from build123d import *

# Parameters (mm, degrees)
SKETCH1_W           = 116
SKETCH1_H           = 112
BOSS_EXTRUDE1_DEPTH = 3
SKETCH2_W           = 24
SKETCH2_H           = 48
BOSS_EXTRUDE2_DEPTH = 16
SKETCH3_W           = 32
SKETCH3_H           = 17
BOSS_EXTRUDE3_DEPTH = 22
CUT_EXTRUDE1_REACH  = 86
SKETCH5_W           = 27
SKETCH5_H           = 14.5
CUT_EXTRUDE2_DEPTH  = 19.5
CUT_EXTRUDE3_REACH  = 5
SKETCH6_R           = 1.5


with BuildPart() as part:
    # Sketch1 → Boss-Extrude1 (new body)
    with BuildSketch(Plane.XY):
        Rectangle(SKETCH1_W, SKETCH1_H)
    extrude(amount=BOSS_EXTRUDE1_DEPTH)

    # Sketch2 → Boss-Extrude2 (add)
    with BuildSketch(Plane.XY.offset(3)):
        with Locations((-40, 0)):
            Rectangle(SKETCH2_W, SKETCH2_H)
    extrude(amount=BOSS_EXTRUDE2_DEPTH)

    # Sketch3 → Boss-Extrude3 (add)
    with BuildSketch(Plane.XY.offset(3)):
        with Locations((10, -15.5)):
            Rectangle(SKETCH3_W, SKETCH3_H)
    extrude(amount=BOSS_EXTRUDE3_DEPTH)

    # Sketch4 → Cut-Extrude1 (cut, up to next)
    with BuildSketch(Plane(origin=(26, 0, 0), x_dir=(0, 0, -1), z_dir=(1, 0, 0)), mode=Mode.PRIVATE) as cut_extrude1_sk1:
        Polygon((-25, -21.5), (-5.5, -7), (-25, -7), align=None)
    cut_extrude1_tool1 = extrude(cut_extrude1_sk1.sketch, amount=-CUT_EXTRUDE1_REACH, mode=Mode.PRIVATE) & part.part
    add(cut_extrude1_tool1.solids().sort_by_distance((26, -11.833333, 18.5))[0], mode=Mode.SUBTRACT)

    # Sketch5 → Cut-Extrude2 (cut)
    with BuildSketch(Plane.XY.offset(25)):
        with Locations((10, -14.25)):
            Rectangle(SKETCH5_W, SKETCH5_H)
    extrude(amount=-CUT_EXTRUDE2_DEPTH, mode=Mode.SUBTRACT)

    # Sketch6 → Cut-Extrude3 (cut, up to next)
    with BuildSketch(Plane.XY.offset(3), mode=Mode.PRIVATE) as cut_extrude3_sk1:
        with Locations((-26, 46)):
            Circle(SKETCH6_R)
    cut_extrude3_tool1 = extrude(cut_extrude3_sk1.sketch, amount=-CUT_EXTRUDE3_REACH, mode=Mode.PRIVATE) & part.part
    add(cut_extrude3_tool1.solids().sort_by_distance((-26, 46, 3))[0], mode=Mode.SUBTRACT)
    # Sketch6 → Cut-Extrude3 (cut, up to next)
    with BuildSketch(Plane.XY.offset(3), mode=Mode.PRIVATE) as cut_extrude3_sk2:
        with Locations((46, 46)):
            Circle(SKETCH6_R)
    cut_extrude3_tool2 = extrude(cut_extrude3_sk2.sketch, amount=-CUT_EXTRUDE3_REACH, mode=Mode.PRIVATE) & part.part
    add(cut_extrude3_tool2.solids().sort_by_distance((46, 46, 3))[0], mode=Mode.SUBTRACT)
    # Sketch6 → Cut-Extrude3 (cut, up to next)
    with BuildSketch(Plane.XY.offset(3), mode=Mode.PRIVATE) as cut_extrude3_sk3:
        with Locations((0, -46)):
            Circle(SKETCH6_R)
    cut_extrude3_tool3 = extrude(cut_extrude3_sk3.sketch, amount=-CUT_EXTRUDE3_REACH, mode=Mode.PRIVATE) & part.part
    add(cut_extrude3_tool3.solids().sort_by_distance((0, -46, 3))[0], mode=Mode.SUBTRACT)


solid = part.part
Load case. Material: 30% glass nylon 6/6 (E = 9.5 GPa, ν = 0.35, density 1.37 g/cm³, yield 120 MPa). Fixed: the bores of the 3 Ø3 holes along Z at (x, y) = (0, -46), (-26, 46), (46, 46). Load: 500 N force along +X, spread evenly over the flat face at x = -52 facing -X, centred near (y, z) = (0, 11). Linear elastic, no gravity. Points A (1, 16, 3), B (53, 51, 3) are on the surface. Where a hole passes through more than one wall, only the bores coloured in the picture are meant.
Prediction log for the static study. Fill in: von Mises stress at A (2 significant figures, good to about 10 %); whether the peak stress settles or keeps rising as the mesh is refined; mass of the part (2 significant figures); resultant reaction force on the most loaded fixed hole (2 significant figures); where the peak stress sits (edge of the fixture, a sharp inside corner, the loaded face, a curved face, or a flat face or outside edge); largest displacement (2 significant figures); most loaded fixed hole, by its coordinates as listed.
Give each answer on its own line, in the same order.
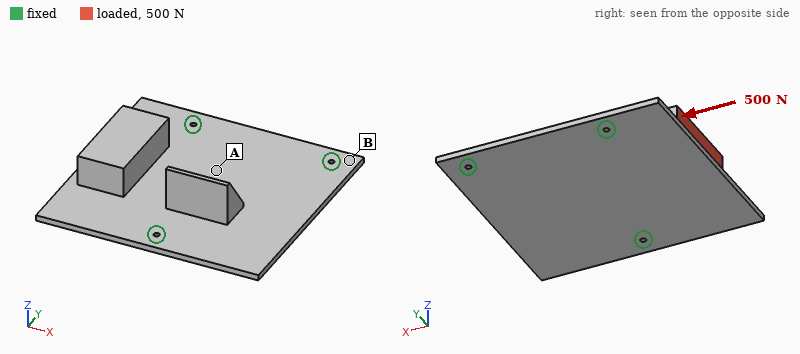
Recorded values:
9.5 MPa
keeps rising
84 g
230 N
edge of the fixture
1.7 mm
(0, -46)
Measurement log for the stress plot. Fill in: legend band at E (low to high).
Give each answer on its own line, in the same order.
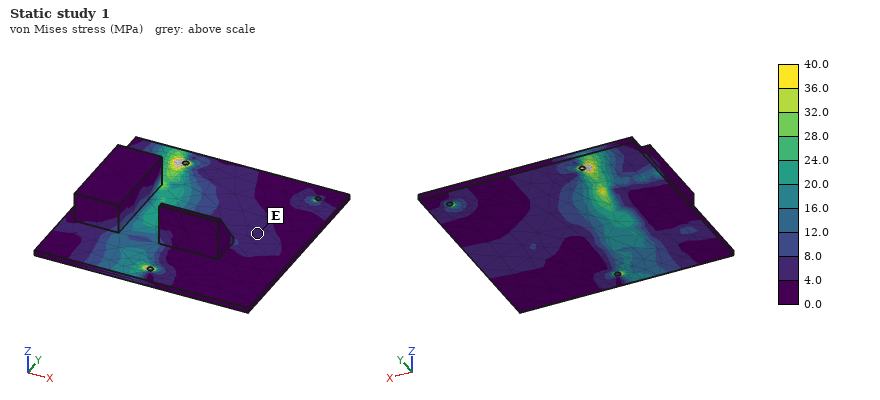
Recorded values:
4.0 to 8.0 MPa
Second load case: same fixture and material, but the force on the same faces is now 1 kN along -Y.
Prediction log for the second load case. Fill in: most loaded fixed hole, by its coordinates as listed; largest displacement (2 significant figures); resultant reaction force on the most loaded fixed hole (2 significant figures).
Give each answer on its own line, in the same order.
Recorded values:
(-26, 46)
1.6 mm
680 N
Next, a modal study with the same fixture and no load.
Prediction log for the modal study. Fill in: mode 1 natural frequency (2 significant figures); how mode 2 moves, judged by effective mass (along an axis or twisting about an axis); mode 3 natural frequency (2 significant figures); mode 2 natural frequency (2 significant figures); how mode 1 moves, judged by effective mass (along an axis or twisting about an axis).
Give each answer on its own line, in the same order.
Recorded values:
300 Hz
along Z
820 Hz
490 Hz
along Z
